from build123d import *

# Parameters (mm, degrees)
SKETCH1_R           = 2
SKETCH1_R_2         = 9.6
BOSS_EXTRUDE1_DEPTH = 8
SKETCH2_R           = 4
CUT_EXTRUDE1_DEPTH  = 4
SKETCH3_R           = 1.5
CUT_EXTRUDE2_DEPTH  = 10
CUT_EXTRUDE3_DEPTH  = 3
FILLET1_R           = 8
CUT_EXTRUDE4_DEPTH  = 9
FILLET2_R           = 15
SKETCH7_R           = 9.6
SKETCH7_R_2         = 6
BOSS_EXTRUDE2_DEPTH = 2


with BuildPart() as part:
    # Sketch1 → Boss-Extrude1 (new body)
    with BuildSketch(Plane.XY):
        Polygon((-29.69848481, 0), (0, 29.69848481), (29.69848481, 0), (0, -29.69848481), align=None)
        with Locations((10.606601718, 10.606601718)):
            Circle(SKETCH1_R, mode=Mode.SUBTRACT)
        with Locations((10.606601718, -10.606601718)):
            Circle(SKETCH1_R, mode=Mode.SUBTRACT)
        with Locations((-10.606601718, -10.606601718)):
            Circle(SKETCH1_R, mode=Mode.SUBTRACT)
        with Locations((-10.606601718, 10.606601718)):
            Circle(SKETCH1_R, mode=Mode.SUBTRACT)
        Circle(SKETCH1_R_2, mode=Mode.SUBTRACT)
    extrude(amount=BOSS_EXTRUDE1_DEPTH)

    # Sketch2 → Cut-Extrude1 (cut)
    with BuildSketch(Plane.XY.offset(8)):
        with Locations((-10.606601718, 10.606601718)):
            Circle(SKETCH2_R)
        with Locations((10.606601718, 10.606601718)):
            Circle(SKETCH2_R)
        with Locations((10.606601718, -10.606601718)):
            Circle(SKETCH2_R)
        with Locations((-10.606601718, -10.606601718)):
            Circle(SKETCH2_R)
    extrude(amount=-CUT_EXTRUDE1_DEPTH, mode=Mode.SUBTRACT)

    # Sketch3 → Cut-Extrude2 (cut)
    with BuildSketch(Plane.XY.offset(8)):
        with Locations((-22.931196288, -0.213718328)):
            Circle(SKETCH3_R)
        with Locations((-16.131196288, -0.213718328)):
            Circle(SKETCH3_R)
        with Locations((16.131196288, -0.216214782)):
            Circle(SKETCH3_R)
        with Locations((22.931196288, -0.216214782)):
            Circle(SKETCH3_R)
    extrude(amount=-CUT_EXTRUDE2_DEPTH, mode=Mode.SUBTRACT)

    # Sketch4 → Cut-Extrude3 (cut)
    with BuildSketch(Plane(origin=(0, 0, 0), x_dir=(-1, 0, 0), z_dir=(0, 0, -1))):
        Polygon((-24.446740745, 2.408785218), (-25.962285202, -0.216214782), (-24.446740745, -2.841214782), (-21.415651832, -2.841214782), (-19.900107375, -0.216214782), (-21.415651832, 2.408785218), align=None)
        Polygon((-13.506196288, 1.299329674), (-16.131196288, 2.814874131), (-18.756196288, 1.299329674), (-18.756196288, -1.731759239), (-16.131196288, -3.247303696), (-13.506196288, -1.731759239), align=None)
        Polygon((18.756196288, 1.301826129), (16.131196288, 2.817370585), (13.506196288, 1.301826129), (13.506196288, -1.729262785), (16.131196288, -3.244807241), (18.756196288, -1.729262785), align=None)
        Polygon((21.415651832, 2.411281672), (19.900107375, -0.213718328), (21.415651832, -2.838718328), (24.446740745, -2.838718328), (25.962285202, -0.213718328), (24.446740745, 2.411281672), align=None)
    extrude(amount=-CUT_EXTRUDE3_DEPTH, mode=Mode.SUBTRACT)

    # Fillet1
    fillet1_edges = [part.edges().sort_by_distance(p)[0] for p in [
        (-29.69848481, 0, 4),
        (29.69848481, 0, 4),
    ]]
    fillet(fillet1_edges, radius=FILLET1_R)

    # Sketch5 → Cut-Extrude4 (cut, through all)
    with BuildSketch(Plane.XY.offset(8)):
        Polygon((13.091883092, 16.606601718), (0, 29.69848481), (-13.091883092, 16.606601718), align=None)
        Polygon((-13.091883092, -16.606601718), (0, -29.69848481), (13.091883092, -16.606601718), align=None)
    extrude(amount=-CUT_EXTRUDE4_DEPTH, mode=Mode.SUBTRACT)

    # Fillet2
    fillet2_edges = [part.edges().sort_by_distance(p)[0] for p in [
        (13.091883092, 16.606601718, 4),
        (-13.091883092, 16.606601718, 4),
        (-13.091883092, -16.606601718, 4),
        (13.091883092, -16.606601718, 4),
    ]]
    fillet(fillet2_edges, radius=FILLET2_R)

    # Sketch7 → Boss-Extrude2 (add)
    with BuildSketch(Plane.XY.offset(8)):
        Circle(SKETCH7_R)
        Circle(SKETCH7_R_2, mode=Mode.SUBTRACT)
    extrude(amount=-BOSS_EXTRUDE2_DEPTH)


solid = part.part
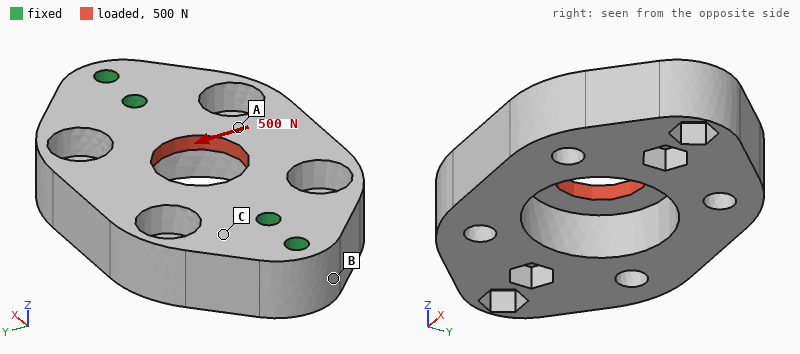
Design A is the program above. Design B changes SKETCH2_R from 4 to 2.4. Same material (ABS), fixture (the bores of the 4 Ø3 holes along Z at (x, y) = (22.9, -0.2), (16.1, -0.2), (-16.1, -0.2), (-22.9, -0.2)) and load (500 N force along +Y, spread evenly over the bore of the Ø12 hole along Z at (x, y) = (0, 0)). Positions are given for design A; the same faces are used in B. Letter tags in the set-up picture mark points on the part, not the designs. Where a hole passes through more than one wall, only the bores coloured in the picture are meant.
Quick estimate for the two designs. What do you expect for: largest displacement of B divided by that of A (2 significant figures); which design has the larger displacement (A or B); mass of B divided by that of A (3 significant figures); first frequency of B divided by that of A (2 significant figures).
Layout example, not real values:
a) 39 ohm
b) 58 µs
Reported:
a) 0.77
b) A
c) 1.07
d) 0.99
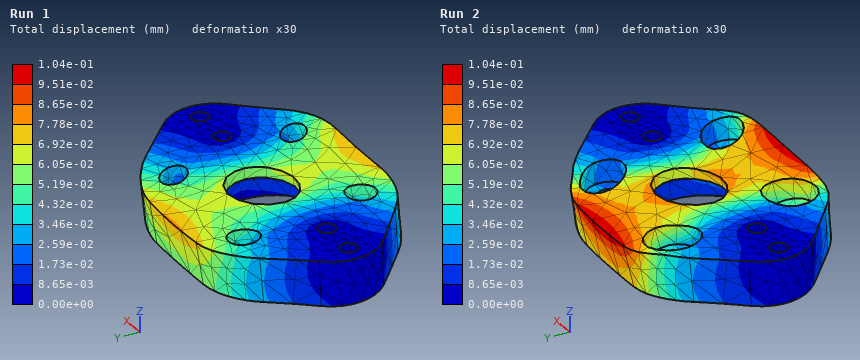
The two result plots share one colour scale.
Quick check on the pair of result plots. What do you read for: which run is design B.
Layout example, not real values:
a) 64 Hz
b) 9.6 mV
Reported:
a) Run 1
